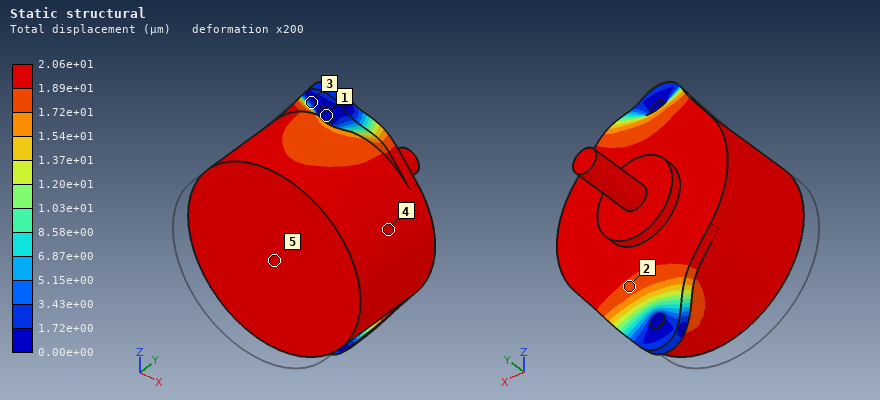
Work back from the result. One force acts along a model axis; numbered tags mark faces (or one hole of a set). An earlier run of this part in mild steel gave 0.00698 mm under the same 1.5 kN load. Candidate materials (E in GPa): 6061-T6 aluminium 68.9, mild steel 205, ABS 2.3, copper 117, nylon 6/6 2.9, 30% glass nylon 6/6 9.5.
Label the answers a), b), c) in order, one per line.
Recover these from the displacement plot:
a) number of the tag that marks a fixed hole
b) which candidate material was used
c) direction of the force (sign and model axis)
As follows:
a) 1
b) 6061-T6 aluminium
c) +Y
